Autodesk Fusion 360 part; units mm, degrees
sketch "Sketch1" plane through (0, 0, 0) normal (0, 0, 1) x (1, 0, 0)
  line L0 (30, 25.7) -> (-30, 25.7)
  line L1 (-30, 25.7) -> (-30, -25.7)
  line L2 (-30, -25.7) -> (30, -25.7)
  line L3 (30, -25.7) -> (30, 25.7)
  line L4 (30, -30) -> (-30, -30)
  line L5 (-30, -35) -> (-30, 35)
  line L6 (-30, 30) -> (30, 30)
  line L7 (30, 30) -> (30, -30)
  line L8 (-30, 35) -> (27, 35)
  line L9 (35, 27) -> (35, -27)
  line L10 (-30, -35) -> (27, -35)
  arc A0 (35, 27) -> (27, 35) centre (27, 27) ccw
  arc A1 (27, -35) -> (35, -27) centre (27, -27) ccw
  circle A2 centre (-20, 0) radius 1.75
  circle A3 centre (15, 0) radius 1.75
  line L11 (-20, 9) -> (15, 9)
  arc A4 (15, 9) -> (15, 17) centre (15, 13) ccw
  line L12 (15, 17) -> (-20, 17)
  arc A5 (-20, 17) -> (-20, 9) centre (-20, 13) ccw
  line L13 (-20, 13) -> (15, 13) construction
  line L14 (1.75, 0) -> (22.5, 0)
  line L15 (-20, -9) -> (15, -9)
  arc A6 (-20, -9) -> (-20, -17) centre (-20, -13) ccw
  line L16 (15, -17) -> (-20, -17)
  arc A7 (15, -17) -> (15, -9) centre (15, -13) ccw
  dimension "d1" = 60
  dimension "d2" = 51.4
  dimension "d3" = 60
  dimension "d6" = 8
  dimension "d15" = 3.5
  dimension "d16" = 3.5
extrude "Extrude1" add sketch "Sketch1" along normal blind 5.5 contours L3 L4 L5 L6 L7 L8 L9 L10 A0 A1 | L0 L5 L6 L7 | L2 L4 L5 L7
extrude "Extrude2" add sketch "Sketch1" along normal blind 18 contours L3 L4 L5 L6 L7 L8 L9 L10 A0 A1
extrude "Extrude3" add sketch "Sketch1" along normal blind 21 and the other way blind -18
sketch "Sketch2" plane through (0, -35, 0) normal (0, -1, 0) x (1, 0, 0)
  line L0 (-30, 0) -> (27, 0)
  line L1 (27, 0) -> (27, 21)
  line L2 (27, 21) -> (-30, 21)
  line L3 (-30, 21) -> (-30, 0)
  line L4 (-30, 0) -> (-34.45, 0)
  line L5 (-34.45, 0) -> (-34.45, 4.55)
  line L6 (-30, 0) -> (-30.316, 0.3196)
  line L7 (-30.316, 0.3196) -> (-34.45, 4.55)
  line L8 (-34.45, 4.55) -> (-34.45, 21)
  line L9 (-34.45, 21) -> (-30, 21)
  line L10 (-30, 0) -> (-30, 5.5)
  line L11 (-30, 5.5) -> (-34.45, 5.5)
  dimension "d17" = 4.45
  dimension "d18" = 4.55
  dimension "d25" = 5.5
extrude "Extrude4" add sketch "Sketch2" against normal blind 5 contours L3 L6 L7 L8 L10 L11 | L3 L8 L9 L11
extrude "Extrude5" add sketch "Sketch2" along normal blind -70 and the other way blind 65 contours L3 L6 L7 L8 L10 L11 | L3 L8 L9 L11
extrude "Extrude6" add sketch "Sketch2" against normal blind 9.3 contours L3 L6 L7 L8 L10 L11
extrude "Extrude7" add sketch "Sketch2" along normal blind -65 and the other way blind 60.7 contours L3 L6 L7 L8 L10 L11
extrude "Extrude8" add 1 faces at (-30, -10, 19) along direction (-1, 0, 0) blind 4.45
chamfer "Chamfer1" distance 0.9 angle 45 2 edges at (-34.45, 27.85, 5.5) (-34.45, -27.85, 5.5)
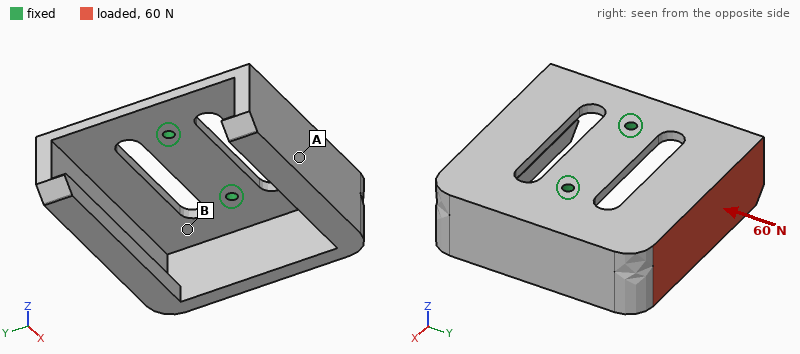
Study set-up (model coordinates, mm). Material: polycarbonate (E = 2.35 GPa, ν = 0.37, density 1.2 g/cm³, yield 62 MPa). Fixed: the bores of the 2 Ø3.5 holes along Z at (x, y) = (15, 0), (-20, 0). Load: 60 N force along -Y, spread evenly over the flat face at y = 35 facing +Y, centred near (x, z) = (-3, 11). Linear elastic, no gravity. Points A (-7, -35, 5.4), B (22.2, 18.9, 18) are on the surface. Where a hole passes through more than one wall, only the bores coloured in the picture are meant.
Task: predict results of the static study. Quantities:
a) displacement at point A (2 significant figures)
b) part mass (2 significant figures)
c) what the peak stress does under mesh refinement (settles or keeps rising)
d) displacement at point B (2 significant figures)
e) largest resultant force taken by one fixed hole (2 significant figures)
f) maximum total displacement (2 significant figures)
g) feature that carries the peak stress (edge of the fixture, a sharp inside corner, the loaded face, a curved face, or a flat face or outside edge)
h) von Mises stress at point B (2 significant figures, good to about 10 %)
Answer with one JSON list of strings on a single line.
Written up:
["0.70 mm", "39 g", "keeps rising", "0.39 mm", "32 N", "1.0 mm", "edge of the fixture", "1.7 MPa"]
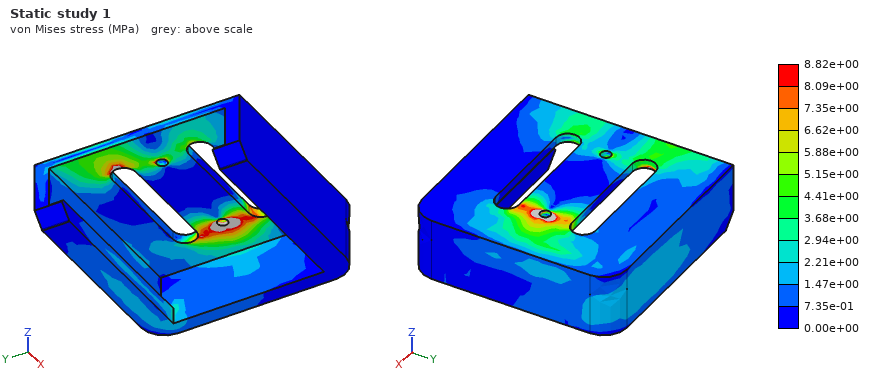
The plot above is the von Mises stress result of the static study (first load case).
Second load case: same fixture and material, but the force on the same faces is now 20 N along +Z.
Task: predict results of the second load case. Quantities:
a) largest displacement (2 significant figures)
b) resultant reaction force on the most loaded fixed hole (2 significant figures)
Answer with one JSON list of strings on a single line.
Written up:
["1.2 mm", "10 N"]
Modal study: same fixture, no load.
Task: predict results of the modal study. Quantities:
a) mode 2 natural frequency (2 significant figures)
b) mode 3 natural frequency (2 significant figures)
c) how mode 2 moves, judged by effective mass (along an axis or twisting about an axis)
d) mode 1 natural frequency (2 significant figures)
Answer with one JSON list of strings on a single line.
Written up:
["350 Hz", "510 Hz", "along Z", "160 Hz"]
